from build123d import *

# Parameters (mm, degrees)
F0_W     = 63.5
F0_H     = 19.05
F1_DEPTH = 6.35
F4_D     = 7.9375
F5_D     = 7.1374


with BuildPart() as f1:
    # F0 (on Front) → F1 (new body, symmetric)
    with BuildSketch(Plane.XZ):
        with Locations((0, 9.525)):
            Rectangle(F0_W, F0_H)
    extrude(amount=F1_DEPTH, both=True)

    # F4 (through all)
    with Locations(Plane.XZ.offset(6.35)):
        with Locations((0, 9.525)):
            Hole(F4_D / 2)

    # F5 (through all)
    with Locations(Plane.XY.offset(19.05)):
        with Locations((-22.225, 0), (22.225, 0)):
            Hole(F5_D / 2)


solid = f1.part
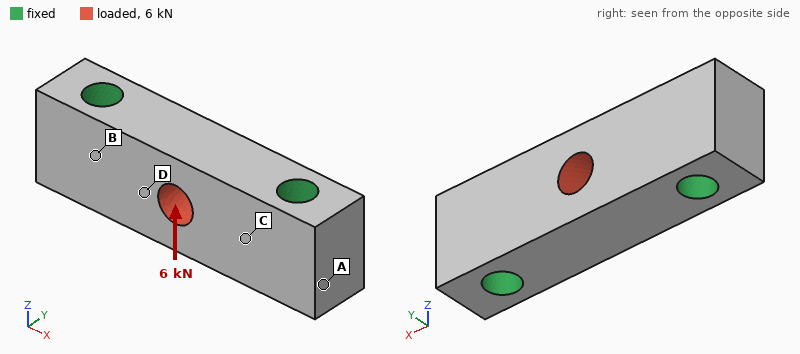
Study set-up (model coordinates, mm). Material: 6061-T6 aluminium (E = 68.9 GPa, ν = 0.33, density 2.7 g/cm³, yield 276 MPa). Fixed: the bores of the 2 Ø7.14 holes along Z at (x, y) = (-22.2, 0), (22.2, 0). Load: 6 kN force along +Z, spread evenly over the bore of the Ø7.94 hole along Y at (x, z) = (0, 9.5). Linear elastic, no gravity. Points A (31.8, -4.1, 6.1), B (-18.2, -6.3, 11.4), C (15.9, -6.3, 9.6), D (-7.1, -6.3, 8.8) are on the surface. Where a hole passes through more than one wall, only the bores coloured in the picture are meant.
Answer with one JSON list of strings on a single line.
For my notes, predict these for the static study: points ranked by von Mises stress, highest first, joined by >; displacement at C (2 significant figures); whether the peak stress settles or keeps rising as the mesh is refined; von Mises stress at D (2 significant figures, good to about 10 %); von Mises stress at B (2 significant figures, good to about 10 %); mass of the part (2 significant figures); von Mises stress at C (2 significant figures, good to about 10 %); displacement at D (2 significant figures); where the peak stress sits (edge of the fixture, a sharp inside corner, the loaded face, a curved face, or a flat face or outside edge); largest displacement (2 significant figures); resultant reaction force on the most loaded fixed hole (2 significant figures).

["D > C > B > A", "2.4 µm", "keeps rising", "33 MPa", "16 MPa", "36 g", "25 MPa", "9.8 µm", "edge of the fixture", "15 µm", "3.0 kN"]
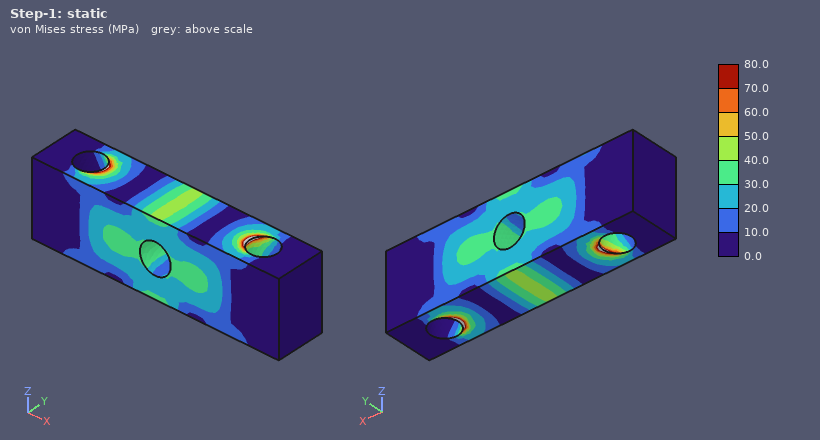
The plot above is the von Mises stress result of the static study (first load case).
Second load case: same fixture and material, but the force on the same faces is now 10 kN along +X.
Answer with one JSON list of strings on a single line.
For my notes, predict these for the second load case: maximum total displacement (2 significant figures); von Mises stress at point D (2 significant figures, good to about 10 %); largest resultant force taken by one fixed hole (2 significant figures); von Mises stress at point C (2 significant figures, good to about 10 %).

["6.8 µm", "32 MPa", "5.0 kN", "15 MPa"]
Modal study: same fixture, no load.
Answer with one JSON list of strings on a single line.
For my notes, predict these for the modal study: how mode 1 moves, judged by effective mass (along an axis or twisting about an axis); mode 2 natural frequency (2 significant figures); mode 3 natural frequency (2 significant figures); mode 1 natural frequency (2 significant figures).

["along Y", "34 kHz", "35 kHz", "25 kHz"]
